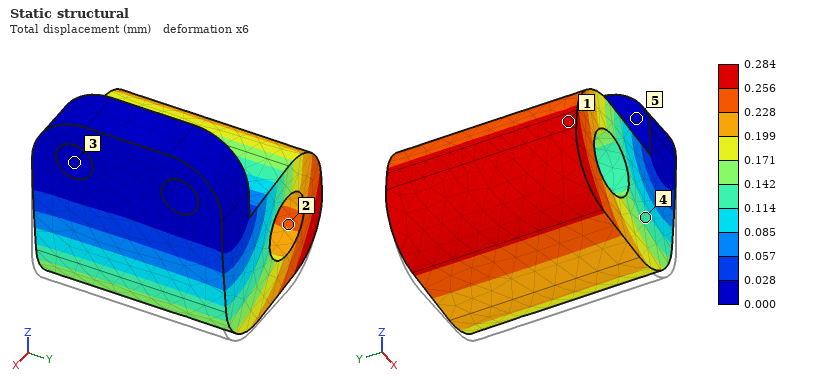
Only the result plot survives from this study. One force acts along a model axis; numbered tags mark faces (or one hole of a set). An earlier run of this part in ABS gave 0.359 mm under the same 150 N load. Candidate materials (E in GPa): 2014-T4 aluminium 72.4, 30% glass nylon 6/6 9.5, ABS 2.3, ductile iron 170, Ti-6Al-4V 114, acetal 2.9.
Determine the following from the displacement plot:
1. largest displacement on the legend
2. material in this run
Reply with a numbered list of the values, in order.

1. 0.284 mm
2. acetal
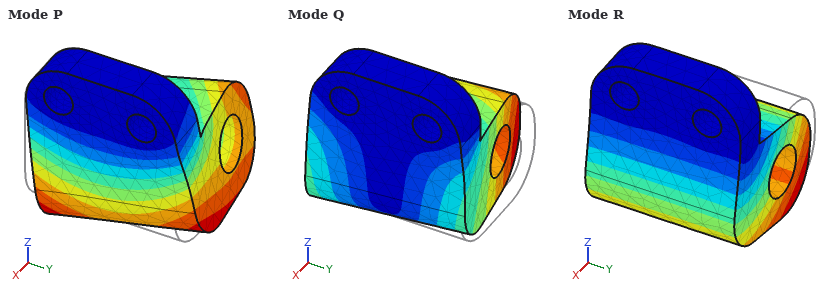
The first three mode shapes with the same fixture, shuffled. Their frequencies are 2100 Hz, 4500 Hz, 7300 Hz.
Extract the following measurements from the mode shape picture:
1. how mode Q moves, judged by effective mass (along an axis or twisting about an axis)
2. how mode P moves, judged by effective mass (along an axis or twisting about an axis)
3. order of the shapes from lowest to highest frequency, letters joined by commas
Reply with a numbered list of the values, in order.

1. along Y
2. along Y
3. R, Q, P
